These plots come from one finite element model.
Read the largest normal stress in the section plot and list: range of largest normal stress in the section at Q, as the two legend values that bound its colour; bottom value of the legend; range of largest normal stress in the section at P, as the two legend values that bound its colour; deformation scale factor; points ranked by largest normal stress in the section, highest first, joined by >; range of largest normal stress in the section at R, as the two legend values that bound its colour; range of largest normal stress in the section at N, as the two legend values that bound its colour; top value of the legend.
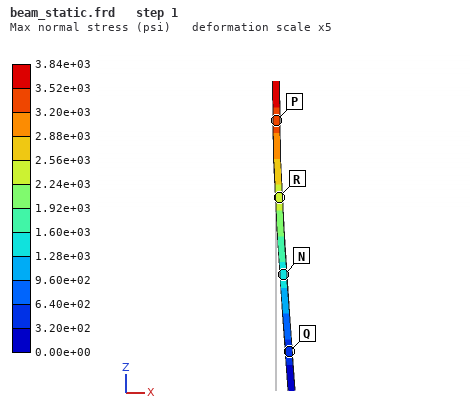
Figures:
3.20e+02 to 6.40e+02 psi
0.00e+00 psi
3.20e+03 to 3.52e+03 psi
5
P > R > N > Q
2.24e+03 to 2.56e+03 psi
1.28e+03 to 1.60e+03 psi
3.84e+03 psi
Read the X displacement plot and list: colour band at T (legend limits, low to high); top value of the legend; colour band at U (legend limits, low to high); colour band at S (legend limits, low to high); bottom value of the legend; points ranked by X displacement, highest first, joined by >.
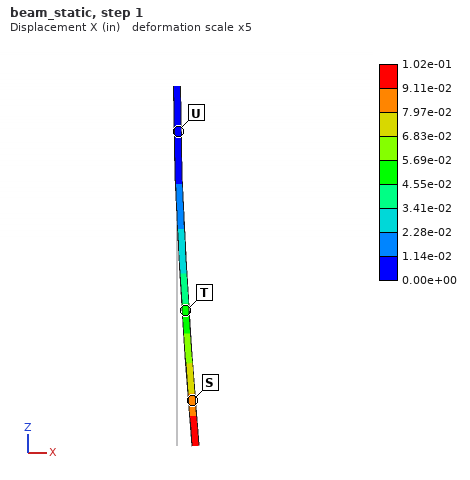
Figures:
4.55e-02 to 5.69e-02 in
1.02e-01 in
0.00e+00 to 1.14e-02 in
7.97e-02 to 9.11e-02 in
0.00e+00 in
S > T > U
